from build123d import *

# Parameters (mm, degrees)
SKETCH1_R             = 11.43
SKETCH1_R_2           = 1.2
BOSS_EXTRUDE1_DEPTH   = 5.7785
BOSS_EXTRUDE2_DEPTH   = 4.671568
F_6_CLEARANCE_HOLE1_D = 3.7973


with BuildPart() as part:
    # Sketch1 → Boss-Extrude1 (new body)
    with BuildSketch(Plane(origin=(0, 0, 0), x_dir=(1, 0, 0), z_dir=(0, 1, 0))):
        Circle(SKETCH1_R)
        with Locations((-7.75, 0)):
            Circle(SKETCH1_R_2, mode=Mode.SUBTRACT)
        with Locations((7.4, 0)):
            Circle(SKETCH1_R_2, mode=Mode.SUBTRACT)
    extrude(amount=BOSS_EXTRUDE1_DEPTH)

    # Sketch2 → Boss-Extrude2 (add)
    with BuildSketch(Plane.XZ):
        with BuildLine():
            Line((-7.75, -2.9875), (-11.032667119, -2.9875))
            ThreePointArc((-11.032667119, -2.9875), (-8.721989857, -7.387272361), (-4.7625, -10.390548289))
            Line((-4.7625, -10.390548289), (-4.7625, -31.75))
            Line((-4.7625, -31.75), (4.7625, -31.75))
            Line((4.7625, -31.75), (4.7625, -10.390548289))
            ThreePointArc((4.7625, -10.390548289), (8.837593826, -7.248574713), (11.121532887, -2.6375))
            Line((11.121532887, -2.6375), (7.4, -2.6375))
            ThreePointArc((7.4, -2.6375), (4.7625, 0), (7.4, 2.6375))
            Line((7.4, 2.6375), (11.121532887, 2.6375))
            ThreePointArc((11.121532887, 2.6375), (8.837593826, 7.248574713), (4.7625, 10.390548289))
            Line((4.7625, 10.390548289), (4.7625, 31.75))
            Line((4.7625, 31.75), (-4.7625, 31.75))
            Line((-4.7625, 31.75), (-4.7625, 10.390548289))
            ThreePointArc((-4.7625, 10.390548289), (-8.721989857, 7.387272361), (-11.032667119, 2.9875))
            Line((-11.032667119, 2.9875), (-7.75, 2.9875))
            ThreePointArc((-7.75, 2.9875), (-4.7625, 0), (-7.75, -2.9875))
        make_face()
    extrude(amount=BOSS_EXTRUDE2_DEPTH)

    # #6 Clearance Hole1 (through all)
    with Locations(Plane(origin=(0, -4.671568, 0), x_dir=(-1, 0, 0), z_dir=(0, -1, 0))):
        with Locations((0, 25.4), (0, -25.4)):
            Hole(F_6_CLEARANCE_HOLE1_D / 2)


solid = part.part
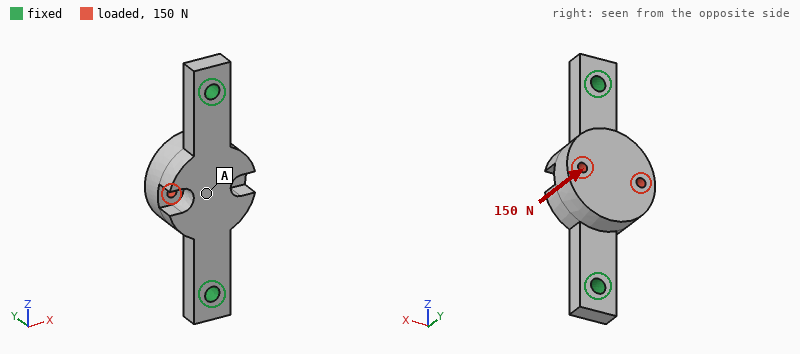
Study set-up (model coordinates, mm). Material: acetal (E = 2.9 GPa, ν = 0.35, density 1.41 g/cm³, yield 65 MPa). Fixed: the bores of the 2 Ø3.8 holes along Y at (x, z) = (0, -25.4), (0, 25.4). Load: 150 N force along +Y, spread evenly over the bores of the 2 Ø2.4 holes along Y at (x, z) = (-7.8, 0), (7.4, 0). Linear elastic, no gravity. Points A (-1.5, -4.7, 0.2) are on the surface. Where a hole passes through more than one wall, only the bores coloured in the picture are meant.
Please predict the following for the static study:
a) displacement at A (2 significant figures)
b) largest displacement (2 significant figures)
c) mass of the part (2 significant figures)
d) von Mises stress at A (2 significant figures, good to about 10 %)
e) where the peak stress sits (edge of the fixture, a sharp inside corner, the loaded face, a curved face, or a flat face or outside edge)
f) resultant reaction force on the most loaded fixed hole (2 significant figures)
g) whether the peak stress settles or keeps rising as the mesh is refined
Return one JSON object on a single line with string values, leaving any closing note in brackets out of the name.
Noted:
{"displacement at A": "0.14 mm", "largest displacement": "0.16 mm", "mass of the part": "8.0 g", "von Mises stress at A": "3.5 MPa", "where the peak stress sits": "edge of the fixture", "resultant reaction force on the most loaded fixed hole": "93 N", "whether the peak stress settles or keeps rising as the mesh is refined": "keeps rising"}
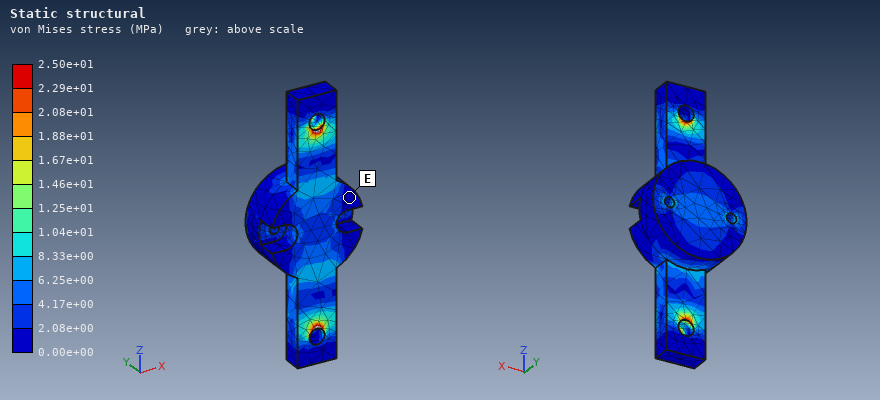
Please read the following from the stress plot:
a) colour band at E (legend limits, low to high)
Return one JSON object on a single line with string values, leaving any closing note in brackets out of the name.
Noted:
{"colour band at E": "0.00e+00 to 2.08e+00 MPa"}
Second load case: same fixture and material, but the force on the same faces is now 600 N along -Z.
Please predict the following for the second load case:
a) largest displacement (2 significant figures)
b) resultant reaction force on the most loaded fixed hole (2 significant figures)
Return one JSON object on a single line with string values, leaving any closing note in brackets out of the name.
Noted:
{"largest displacement": "0.12 mm", "resultant reaction force on the most loaded fixed hole": "310 N"}
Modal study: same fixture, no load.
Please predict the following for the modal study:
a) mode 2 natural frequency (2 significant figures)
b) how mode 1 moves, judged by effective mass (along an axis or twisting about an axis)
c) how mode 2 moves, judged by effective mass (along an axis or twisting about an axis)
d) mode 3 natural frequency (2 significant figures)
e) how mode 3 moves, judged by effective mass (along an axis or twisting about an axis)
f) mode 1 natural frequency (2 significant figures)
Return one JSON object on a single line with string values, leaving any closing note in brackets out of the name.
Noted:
{"mode 2 natural frequency": "2200 Hz", "how mode 1 moves, judged by effective mass": "along X", "how mode 2 moves, judged by effective mass": "along Y", "mode 3 natural frequency": "3400 Hz", "how mode 3 moves, judged by effective mass": "along X", "mode 1 natural frequency": "1700 Hz"}
